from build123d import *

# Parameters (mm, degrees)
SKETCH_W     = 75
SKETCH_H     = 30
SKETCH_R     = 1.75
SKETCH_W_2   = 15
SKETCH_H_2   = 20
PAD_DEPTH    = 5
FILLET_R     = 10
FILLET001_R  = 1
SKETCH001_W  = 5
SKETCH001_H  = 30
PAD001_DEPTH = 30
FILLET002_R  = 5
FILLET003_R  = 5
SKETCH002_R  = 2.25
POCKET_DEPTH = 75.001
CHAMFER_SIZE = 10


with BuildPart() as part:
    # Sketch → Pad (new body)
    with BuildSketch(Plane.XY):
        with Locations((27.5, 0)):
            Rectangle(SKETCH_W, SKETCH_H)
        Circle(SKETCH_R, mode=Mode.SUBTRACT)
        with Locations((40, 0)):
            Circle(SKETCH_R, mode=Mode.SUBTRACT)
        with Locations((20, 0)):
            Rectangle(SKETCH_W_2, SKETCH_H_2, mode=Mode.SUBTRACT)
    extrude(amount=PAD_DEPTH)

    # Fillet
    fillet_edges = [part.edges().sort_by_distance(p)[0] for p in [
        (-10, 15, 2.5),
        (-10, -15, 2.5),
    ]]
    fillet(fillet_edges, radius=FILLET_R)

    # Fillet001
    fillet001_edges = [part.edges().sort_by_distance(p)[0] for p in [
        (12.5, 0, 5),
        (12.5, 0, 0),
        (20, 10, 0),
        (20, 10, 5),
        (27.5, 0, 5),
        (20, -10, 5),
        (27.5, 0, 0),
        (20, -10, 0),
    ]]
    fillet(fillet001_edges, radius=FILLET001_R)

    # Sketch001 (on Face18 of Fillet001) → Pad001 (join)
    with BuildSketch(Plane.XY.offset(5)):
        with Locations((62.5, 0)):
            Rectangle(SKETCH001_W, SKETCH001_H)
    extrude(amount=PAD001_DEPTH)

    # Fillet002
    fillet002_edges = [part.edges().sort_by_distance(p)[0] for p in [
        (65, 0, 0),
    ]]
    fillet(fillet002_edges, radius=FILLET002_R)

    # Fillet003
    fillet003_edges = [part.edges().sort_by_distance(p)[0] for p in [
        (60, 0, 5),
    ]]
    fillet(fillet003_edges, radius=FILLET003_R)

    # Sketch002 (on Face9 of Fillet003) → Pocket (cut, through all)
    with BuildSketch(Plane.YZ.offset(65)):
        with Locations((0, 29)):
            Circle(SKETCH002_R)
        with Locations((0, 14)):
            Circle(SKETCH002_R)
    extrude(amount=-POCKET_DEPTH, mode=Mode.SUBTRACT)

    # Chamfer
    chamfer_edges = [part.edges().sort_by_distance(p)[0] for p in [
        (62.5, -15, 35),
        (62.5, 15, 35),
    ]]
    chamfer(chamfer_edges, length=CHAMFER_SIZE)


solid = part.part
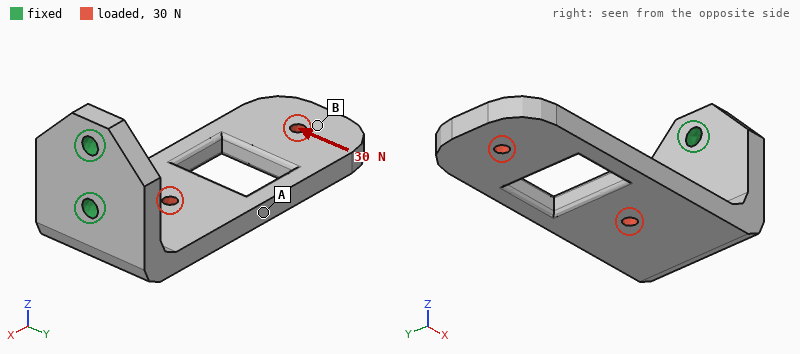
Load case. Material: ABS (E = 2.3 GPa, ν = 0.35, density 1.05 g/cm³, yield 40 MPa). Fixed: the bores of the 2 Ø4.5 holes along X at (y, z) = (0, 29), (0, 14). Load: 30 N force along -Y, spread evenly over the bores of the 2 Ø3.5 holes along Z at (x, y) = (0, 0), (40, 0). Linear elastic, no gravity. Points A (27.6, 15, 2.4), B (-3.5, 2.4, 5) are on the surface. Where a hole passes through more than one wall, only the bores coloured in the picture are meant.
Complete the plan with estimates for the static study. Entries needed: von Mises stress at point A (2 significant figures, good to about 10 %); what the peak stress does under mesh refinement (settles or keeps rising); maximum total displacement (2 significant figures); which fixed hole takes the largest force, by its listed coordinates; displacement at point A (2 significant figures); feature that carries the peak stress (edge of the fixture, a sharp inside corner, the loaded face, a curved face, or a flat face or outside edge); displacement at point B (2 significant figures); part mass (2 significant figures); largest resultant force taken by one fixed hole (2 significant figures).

2.9 MPa
keeps rising
0.91 mm
(0, 14)
0.44 mm
edge of the fixture
0.83 mm
14 g
45 N
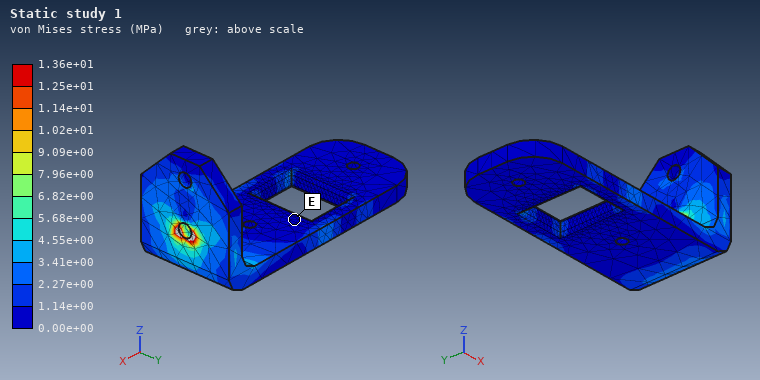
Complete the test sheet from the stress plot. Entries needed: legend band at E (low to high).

0.00e+00 to 1.14e+00 MPa
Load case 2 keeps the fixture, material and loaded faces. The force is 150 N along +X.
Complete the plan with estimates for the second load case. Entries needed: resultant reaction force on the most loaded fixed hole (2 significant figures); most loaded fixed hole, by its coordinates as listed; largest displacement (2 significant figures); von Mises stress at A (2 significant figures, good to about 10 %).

190 N
(0, 14)
1.1 mm
1.5 MPa
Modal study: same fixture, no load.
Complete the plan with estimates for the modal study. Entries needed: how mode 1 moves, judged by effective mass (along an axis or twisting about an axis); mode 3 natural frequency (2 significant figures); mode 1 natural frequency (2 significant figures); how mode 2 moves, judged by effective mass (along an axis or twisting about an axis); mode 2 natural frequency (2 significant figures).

along Z
990 Hz
210 Hz
along Y
400 Hz
